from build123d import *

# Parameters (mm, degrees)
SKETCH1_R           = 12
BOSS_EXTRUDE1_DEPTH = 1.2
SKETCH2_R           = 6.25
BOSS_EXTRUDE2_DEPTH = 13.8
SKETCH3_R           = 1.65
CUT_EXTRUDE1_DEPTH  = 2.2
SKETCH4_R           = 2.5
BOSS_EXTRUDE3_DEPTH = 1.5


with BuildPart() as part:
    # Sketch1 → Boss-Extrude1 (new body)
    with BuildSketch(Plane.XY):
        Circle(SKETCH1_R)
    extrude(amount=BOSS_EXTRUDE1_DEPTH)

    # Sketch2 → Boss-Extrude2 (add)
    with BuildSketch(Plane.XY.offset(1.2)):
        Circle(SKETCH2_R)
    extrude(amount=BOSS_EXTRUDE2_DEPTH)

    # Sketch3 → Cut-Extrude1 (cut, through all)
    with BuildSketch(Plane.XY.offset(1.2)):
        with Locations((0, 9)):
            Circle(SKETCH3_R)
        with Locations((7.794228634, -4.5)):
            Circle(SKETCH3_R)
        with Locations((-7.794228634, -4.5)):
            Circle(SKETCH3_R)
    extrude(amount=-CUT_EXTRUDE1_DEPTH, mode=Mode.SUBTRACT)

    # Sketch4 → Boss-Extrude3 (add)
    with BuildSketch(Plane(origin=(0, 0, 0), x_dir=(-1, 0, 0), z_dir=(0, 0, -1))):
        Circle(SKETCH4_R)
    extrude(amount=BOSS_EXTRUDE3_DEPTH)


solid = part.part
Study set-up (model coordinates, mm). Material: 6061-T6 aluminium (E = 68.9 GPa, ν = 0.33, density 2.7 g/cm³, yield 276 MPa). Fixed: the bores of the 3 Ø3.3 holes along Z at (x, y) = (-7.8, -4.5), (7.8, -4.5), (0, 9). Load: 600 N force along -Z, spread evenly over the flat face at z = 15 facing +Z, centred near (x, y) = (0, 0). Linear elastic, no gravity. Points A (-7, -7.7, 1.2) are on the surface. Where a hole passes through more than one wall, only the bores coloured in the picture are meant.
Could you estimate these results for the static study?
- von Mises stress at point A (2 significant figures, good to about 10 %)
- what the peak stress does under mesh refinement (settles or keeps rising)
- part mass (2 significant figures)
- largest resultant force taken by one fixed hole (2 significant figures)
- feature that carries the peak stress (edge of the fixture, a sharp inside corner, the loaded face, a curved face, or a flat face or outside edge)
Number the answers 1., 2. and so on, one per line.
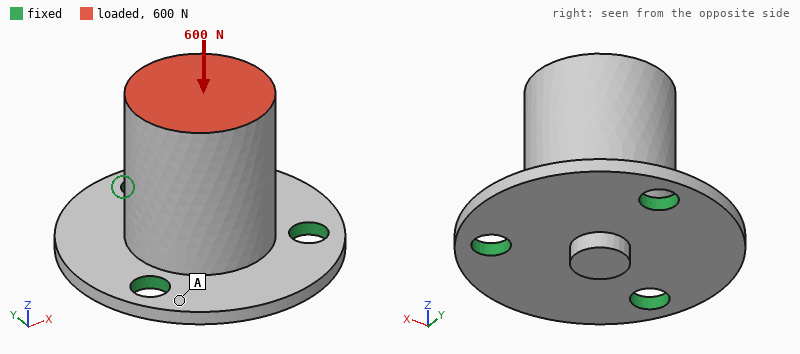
1. 13 MPa
2. keeps rising
3. 6.0 g
4. 220 N
5. edge of the fixture
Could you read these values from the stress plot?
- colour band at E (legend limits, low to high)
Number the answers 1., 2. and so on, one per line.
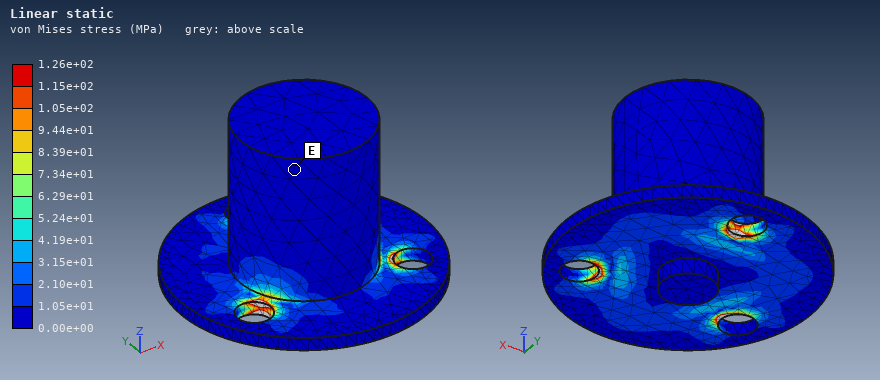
1. 0.00e+00 to 1.05e+01 MPa
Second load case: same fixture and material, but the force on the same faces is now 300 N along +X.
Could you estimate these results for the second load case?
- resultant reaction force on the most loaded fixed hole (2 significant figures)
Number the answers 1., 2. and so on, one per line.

1. 370 N
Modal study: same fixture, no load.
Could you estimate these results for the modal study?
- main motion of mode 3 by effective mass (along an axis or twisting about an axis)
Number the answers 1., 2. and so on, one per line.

1. along Z
